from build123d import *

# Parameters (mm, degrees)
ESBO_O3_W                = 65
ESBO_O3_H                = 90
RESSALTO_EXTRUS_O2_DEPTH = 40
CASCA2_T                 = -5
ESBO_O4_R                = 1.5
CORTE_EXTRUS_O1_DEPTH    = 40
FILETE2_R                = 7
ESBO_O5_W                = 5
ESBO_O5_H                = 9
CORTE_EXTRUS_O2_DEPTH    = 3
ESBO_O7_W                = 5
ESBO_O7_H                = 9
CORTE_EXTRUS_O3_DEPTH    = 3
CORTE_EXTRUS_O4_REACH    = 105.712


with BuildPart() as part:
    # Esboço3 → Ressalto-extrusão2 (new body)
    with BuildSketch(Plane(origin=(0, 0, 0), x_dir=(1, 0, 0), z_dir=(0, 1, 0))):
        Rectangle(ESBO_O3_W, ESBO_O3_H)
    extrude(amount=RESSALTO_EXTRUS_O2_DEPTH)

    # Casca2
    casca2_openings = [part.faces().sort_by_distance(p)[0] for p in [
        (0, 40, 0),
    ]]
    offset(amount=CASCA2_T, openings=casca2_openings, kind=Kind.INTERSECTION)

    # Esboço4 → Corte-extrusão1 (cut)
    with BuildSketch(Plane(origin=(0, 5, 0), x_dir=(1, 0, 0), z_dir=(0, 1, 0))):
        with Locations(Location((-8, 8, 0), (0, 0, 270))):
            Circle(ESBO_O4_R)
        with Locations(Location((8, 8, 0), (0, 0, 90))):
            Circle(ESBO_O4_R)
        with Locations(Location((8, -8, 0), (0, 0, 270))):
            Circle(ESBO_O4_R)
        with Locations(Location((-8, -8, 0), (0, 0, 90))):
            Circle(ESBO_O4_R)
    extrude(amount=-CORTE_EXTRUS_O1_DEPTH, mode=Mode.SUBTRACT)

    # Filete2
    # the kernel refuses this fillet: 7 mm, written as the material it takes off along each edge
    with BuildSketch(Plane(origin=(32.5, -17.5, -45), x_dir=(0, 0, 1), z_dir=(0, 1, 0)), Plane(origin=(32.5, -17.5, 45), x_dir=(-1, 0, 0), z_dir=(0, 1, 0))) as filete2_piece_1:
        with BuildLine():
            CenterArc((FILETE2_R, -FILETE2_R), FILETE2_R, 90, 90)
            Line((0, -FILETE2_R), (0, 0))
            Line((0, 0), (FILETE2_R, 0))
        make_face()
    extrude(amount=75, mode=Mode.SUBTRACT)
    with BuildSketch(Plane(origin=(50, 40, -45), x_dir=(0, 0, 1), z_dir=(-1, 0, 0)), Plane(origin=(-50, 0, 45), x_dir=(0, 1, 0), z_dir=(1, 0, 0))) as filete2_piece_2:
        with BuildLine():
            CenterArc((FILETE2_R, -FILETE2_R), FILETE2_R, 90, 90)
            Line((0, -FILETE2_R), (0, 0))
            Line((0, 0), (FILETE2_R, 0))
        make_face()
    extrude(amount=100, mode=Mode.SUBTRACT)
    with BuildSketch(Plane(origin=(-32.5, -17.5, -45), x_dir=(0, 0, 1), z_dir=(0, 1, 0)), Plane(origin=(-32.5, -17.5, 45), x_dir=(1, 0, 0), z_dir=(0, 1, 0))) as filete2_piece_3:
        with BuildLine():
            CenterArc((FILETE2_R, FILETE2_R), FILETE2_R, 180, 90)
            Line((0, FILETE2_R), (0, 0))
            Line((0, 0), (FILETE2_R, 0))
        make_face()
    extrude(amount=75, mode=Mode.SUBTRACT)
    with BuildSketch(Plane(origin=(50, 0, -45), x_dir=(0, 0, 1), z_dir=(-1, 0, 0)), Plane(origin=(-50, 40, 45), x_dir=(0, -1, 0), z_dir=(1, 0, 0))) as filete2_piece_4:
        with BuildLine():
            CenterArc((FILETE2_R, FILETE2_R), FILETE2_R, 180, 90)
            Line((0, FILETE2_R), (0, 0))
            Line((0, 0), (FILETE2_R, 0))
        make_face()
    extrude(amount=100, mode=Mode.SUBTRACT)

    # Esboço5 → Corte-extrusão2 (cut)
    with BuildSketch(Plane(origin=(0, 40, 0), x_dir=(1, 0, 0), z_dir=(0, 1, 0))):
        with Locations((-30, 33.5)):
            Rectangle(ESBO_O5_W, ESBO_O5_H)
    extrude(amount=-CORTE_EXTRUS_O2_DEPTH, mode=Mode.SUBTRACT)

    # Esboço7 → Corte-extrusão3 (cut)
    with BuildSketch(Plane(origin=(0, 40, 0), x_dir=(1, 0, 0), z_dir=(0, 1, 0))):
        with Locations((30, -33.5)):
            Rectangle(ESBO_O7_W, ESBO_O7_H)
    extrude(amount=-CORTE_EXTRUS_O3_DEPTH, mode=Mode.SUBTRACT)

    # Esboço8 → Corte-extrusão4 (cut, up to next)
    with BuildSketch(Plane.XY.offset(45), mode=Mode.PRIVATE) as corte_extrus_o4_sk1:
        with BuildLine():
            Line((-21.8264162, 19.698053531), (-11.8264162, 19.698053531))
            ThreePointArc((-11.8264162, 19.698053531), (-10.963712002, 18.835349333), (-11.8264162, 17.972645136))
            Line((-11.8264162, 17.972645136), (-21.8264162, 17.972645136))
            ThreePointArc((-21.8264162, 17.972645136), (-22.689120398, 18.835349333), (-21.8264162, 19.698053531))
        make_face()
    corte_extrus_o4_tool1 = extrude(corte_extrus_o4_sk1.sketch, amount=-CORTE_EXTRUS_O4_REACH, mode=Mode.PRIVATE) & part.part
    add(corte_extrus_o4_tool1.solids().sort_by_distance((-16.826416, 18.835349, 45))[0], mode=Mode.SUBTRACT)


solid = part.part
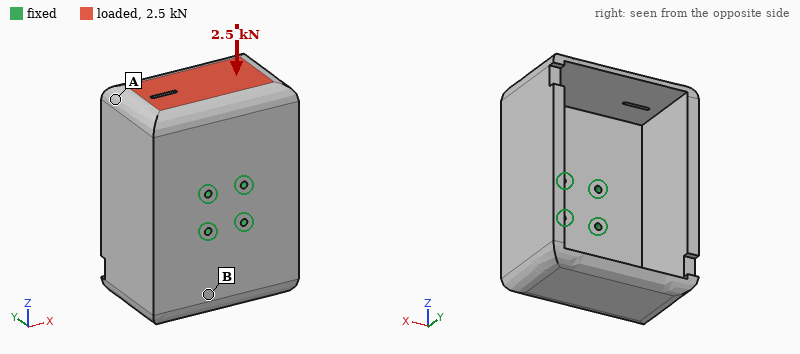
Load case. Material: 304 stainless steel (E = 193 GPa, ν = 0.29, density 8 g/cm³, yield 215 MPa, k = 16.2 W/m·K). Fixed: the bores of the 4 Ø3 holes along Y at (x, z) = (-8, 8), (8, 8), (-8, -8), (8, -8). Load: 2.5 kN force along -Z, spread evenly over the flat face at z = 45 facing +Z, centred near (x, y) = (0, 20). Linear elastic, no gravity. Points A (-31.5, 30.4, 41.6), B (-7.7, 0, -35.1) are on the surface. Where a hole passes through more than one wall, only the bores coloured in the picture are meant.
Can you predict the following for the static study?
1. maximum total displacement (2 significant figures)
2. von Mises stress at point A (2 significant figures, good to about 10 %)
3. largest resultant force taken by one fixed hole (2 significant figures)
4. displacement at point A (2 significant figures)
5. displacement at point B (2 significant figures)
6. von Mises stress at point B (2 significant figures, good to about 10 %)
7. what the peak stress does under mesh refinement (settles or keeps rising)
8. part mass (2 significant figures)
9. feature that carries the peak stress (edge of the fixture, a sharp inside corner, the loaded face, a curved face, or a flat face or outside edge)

91 µm
32 MPa
1.2 kN
54 µm
33 µm
14 MPa
keeps rising
600 g
edge of the fixture
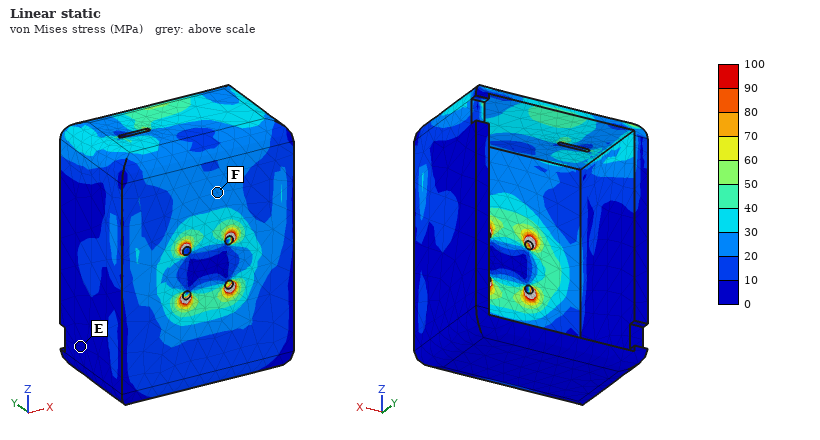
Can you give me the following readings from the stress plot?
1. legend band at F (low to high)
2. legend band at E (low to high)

20 to 30 MPa
0 to 10 MPa
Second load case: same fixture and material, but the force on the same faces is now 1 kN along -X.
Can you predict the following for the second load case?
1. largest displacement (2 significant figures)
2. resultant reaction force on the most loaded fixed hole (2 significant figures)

41 µm
1.3 kN
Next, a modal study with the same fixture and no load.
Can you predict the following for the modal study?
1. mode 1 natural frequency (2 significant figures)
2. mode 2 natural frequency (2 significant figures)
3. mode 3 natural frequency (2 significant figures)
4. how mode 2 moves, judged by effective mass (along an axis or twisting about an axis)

1300 Hz
1500 Hz
1900 Hz
along X
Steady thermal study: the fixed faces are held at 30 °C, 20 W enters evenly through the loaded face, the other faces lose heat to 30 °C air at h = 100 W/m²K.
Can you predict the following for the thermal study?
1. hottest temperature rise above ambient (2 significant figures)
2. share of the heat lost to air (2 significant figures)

44 K
93 %
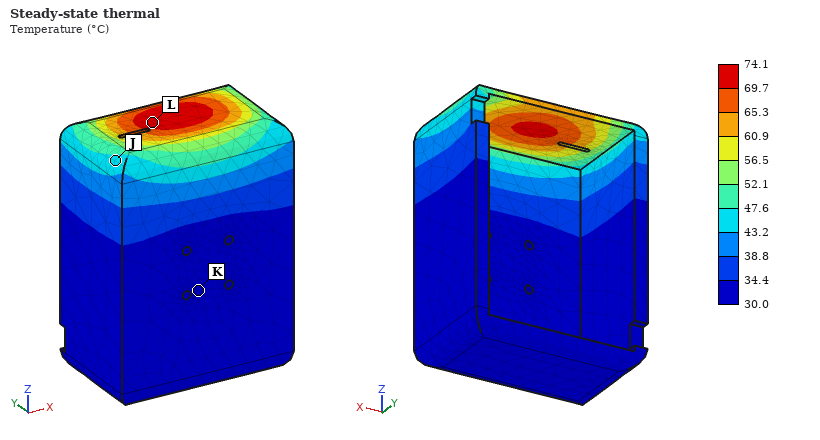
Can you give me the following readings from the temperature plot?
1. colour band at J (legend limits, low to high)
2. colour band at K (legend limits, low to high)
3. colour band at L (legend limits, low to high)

43.2 to 47.6 °C
30.0 to 34.4 °C
69.7 to 74.1 °C
